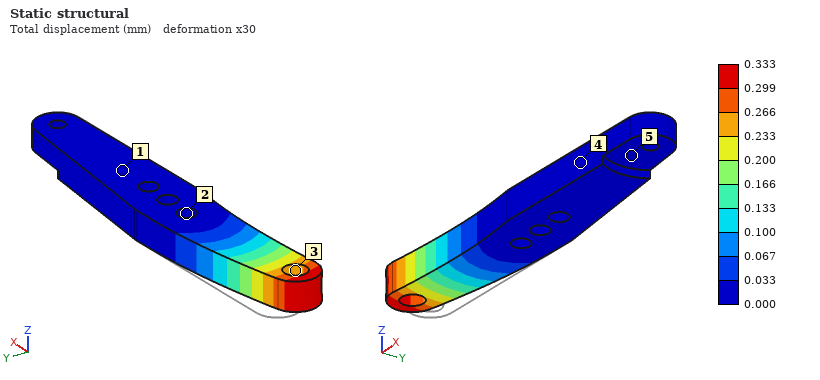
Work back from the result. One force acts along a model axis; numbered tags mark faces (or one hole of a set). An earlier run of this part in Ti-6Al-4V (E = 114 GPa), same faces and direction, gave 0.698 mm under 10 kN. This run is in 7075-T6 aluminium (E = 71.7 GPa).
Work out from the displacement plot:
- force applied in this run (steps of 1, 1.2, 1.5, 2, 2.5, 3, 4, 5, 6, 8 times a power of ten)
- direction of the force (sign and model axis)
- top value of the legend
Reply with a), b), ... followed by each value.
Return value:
a) 3 kN
b) -Y
c) 0.333 mm
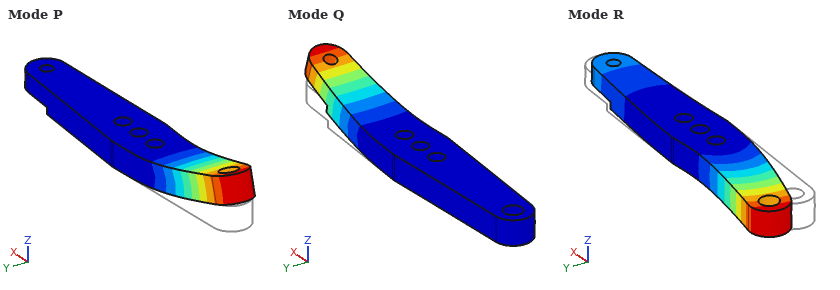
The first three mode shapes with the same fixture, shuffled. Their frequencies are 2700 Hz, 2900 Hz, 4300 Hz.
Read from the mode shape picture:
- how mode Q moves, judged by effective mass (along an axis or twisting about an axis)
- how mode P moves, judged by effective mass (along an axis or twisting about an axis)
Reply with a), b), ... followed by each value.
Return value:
a) along Z
b) along Z
